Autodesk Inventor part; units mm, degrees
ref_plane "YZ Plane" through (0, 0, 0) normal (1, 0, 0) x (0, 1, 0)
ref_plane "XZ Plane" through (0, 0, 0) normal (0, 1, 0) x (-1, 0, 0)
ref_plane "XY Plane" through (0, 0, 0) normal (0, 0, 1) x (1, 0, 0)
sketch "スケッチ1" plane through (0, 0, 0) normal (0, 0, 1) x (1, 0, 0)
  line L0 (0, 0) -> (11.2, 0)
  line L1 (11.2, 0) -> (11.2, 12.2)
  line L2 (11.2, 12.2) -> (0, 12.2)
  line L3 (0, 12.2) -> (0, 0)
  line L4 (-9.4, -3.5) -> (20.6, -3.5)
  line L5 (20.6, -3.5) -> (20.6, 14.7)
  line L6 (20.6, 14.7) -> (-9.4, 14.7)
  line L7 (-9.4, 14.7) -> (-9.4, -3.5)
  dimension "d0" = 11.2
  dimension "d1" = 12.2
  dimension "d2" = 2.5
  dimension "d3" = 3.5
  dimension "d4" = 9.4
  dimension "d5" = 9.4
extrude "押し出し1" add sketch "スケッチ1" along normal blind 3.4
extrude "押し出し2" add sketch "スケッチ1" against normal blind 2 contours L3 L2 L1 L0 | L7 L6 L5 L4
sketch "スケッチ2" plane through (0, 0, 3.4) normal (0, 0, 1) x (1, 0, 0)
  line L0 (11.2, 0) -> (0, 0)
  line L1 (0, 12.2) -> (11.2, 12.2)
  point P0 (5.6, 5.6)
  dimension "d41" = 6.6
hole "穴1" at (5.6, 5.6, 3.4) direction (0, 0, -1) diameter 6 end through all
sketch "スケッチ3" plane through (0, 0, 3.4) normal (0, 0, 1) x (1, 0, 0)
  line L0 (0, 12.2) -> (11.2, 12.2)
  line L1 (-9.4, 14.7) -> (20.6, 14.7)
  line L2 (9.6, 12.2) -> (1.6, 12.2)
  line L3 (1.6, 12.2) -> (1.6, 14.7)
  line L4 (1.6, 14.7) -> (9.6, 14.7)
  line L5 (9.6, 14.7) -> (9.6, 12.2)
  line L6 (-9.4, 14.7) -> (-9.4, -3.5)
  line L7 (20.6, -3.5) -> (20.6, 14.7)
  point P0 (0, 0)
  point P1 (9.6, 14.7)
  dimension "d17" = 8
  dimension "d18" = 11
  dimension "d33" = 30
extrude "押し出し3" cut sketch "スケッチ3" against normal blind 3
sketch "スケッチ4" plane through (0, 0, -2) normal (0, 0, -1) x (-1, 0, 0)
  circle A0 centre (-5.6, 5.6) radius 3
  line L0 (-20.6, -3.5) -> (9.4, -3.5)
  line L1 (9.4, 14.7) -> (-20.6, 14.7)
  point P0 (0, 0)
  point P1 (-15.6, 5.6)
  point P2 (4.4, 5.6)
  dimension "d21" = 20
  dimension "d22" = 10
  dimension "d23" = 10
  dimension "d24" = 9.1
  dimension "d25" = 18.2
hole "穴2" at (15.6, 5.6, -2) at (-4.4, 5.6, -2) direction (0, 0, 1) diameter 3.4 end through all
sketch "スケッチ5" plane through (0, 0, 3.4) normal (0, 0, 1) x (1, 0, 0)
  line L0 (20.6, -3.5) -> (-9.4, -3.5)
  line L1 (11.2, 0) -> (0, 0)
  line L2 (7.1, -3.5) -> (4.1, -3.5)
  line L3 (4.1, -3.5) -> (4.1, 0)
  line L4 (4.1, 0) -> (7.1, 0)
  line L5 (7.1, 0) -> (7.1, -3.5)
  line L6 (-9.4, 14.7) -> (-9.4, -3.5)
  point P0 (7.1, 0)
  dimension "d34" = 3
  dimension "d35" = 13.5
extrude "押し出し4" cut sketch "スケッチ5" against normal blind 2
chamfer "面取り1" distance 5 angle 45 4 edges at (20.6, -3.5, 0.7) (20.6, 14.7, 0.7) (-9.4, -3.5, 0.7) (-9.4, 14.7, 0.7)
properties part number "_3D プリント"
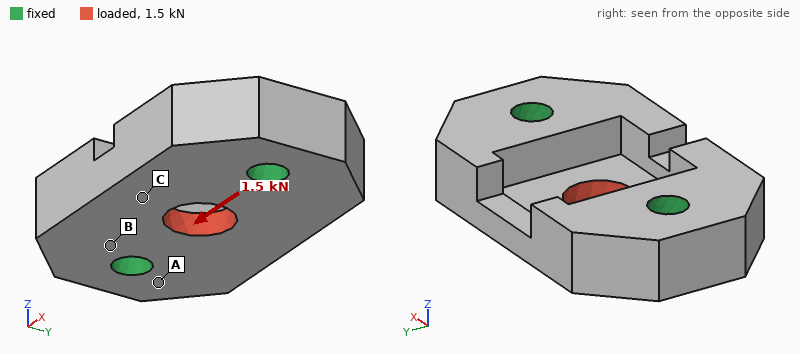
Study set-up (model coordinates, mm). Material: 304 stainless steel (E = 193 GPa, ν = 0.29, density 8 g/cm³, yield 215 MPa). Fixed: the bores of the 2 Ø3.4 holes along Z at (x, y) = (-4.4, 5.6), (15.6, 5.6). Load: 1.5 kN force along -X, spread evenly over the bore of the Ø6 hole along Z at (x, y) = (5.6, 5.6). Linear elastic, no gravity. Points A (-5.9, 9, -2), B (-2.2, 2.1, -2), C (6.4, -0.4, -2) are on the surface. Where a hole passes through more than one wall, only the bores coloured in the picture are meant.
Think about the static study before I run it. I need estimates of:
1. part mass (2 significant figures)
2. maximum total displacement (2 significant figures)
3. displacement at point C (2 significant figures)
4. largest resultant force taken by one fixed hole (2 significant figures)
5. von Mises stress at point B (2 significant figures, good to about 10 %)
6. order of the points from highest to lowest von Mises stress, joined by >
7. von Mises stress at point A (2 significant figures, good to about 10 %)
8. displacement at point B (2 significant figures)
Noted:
16 g
1.7 µm
0.69 µm
750 N
19 MPa
B > A > C
11 MPa
0.52 µm
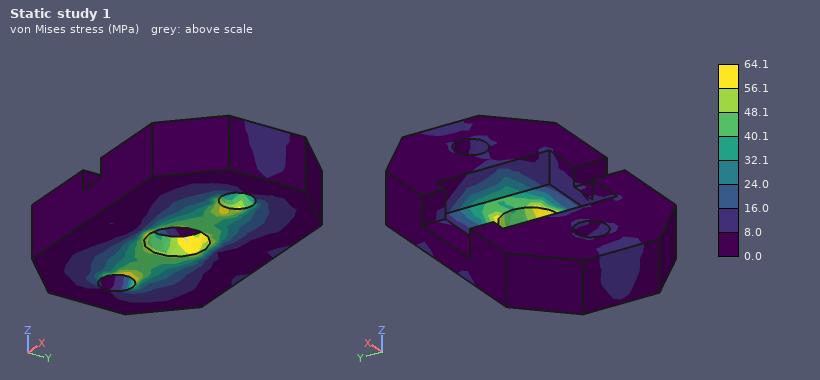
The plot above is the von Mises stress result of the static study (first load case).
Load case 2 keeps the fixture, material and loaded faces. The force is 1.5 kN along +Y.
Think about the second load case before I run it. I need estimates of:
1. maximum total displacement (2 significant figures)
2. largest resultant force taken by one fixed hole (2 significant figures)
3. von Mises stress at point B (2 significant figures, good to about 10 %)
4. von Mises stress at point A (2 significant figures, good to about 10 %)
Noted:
3.1 µm
750 N
32 MPa
7.2 MPa
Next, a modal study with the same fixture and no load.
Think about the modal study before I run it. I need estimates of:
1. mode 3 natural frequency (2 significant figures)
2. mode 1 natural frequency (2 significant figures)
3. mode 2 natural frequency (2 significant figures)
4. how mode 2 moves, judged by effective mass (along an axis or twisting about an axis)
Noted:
50 kHz
34 kHz
39 kHz
along Z
